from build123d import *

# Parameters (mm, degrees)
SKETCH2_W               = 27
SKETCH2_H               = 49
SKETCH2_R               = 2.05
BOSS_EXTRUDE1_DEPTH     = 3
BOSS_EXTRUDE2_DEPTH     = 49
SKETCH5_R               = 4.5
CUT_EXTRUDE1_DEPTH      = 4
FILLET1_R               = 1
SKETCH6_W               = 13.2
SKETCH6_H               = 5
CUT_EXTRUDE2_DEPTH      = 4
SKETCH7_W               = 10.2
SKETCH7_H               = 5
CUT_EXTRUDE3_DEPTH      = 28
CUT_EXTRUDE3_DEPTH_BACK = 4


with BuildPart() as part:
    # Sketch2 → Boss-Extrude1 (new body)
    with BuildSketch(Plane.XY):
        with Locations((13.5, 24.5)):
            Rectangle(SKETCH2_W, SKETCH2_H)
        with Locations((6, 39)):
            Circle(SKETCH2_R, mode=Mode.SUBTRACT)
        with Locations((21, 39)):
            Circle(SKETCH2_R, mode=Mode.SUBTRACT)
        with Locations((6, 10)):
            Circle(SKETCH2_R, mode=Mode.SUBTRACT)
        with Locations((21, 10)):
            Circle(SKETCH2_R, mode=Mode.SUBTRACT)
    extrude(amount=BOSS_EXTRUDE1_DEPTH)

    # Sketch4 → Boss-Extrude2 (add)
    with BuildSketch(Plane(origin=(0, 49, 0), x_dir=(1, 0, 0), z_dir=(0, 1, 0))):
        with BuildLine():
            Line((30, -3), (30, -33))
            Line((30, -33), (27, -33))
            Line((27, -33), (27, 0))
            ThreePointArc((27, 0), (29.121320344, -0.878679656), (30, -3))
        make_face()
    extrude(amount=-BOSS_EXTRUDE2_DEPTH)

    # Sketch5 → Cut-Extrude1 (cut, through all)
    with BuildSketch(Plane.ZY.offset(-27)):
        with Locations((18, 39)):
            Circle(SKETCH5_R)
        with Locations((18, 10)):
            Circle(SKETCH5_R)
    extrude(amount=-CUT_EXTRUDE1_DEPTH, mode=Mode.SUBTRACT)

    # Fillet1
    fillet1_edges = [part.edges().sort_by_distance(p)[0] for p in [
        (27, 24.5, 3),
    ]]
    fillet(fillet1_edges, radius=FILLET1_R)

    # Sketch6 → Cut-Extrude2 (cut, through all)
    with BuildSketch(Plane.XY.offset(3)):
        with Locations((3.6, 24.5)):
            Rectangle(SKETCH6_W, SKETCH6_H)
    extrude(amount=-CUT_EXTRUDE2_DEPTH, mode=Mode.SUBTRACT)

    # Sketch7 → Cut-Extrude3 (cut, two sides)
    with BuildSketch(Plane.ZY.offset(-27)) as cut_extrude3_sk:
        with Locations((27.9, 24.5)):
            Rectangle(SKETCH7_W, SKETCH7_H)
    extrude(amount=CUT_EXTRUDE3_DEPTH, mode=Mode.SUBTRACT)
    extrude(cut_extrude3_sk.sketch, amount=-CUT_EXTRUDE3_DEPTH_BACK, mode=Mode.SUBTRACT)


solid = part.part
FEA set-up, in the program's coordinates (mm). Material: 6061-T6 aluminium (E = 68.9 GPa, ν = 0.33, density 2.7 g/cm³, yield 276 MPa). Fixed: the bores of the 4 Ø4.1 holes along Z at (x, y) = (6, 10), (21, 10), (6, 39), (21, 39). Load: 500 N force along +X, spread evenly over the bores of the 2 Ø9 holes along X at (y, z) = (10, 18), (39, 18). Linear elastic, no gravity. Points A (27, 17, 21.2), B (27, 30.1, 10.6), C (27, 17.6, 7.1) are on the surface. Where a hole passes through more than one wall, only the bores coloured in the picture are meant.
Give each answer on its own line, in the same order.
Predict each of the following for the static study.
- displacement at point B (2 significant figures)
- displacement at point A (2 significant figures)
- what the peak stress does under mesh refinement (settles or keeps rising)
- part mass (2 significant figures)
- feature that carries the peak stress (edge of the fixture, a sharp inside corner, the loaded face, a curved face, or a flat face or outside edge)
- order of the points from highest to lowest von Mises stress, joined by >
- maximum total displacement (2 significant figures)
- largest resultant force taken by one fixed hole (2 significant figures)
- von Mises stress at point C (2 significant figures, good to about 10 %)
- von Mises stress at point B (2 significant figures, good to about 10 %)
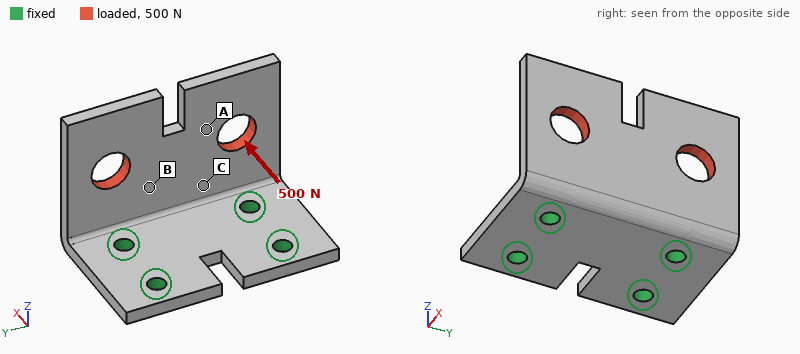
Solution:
0.091 mm
0.24 mm
keeps rising
21 g
edge of the fixture
C > B > A
0.43 mm
220 N
68 MPa
49 MPa
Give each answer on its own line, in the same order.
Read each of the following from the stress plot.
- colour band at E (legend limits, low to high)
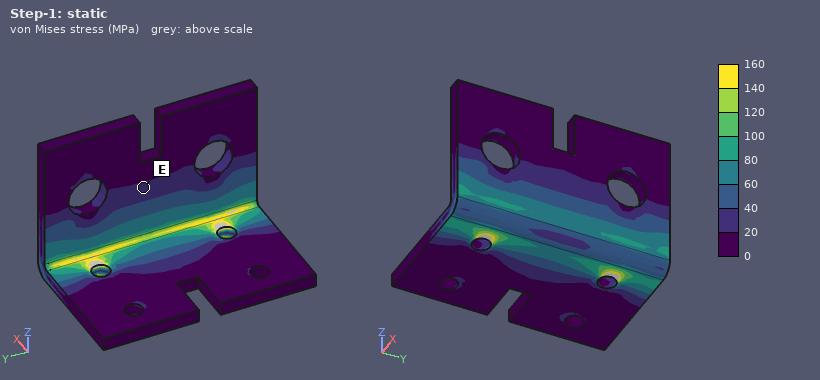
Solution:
20 to 40 MPa
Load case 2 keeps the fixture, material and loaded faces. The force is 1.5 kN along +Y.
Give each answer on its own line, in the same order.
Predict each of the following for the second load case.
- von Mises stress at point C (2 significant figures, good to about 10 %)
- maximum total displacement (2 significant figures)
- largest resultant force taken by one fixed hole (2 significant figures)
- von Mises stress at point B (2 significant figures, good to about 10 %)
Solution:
54 MPa
0.12 mm
1.1 kN
44 MPa
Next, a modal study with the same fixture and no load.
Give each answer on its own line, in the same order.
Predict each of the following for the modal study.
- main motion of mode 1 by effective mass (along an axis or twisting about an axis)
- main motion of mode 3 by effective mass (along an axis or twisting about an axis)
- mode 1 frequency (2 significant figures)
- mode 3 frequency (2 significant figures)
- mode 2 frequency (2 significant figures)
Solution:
along X
along Y
2000 Hz
7500 Hz
3300 Hz
